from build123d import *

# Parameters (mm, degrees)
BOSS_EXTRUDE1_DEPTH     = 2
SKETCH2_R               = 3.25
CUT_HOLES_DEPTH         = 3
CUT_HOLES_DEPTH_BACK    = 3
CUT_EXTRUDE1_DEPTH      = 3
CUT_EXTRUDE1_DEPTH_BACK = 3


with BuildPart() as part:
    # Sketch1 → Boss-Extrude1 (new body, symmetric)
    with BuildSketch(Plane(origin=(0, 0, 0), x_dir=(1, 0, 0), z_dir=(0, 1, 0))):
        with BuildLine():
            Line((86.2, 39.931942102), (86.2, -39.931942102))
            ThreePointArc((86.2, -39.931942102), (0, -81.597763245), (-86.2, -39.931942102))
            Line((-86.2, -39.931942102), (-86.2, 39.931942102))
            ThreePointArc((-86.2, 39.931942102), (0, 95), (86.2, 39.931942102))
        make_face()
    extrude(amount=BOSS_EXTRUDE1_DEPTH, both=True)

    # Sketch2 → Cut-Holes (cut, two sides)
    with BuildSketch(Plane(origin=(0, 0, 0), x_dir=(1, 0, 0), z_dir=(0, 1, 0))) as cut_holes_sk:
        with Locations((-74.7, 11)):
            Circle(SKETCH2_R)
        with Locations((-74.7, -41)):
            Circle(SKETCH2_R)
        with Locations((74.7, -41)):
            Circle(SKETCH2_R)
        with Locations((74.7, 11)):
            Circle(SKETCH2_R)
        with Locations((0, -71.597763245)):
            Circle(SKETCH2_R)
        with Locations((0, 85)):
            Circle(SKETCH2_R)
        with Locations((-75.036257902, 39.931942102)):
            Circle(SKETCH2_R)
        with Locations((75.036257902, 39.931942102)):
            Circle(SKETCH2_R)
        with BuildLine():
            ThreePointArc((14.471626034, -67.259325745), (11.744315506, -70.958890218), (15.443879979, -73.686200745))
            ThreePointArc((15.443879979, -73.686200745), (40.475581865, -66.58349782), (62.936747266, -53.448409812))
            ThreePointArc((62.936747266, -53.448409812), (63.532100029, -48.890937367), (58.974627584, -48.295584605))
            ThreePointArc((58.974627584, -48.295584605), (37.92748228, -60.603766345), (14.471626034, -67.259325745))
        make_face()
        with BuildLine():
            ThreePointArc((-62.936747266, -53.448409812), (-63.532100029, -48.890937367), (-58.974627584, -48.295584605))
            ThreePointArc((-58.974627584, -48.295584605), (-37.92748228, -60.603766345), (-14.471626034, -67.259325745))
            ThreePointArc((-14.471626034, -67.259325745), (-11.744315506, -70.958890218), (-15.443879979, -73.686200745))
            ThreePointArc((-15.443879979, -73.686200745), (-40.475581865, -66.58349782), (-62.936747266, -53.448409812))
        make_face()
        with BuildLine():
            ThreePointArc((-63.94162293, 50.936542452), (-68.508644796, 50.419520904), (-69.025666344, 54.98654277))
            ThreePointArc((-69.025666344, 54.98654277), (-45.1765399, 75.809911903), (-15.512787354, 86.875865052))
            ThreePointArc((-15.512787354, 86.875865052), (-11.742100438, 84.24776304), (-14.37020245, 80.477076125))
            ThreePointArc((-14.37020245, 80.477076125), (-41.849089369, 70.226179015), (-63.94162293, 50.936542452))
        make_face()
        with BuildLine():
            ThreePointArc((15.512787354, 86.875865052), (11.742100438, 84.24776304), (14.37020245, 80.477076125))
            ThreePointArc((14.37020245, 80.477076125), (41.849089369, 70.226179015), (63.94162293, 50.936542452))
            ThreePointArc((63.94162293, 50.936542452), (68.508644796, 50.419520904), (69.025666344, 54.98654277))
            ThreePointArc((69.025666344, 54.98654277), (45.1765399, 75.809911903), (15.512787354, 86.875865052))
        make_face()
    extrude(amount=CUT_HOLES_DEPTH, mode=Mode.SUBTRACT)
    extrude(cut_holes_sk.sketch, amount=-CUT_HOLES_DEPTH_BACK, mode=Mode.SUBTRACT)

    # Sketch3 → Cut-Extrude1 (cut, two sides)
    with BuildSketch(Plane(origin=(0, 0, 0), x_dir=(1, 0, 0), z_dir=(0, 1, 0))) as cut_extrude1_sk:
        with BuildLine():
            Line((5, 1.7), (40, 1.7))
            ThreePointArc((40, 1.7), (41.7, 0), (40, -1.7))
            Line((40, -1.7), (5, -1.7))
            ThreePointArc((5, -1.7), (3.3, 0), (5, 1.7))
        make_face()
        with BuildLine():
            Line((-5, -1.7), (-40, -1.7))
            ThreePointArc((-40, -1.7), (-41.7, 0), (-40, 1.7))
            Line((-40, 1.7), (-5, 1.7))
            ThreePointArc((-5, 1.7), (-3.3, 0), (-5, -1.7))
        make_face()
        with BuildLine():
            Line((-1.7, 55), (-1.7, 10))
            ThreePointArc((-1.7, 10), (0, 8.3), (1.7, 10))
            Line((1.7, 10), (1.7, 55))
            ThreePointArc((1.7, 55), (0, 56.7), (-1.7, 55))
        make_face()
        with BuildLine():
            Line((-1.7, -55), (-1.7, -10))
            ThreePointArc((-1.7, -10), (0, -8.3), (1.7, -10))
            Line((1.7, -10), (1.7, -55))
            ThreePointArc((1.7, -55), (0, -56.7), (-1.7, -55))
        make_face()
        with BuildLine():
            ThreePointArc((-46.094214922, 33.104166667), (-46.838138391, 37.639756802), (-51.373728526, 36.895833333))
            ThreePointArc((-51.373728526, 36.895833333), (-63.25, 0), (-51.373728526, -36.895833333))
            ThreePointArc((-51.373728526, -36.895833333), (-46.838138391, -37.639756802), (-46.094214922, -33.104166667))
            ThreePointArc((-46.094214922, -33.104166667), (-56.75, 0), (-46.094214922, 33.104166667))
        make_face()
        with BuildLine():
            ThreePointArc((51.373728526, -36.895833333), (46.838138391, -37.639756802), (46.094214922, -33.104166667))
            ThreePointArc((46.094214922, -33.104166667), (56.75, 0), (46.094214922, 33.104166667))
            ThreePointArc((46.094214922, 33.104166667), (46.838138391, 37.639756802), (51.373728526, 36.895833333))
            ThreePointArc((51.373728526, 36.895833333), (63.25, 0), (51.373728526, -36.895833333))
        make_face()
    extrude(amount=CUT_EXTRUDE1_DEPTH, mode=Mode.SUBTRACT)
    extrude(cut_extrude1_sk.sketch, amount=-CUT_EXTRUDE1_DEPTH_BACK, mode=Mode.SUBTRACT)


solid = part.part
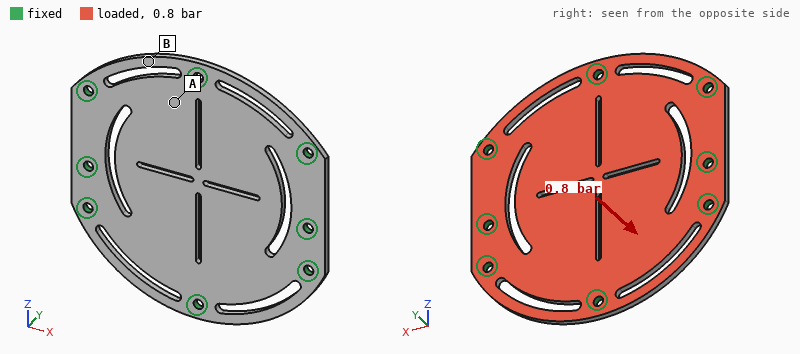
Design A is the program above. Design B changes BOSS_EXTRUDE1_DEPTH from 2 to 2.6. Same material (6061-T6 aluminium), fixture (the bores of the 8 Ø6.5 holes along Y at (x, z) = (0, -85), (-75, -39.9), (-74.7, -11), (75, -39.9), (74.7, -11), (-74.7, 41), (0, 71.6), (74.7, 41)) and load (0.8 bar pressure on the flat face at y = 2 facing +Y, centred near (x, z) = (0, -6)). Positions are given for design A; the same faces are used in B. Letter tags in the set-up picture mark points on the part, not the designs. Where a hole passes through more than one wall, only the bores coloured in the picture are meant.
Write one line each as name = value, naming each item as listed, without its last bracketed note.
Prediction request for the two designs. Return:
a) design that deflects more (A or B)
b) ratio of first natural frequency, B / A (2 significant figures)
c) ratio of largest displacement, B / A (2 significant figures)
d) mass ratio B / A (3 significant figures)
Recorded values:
design that deflects more = A
ratio of first natural frequency, B / A = 1.3
ratio of largest displacement, B / A = 0.47
mass ratio B / A = 1.30
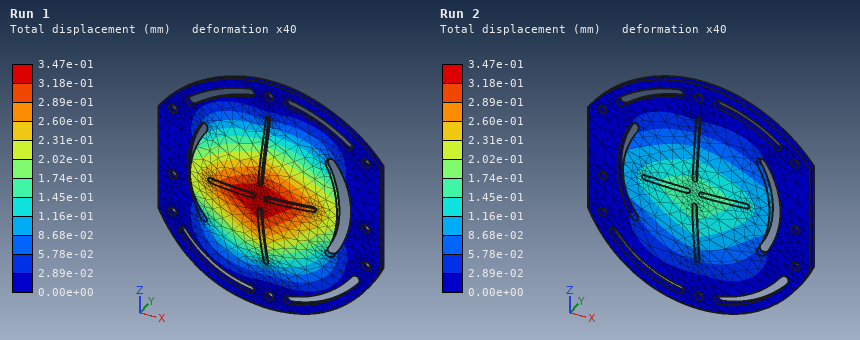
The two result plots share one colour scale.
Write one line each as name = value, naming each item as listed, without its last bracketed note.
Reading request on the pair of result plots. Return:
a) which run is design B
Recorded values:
which run is design B = Run 2
